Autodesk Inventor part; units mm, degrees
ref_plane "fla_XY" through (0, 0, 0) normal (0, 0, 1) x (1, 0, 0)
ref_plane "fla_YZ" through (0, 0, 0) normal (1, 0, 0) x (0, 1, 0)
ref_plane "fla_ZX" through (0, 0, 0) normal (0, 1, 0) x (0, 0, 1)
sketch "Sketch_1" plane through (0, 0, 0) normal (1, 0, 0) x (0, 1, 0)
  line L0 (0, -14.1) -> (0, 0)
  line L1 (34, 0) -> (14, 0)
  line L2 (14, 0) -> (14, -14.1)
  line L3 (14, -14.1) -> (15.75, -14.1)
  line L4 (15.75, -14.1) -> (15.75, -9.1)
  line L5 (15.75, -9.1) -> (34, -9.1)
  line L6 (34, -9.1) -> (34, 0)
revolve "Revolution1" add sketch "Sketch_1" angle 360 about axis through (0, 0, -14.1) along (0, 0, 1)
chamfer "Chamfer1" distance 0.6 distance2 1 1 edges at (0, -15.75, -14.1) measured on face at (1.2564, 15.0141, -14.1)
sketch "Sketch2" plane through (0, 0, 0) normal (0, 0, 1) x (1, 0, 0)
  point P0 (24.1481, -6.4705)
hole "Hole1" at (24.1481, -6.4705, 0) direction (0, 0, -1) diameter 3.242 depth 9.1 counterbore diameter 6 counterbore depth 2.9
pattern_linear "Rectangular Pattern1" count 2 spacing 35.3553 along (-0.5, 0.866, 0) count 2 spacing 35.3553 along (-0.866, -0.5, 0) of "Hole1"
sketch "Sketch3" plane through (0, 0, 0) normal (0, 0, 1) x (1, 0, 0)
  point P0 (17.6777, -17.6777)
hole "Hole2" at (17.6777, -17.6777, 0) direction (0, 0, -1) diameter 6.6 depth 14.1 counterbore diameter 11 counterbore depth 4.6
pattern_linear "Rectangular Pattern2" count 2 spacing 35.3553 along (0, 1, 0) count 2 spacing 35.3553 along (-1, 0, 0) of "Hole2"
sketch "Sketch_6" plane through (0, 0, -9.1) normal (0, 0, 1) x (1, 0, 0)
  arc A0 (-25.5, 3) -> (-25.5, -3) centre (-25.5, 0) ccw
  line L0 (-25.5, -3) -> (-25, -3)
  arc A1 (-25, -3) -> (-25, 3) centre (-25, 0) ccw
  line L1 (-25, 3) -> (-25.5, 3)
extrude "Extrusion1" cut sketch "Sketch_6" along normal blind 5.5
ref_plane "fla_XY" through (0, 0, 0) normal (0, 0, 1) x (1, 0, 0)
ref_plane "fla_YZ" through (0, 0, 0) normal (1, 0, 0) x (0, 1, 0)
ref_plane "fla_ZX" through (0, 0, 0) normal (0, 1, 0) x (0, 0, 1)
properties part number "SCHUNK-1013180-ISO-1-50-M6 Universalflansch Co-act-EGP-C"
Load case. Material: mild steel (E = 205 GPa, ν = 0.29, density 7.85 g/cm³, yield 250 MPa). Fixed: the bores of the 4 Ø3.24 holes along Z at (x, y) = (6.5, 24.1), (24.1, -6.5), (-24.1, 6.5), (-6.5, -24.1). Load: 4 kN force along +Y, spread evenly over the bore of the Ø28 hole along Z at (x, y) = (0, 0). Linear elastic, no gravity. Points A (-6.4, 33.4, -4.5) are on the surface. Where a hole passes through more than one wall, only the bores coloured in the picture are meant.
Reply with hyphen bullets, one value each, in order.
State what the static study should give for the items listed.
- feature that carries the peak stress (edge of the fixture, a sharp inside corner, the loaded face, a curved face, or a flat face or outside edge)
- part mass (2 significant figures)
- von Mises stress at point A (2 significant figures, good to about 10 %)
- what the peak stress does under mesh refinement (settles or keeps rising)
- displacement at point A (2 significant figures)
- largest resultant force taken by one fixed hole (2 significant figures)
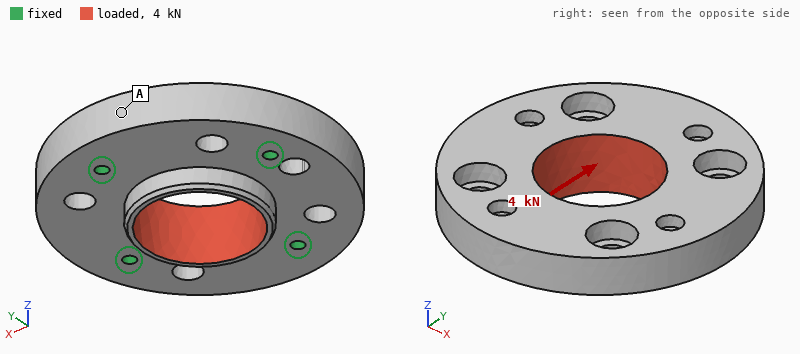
- edge of the fixture
- 200 g
- 3.6 MPa
- keeps rising
- 0.70 µm
- 1.1 kN
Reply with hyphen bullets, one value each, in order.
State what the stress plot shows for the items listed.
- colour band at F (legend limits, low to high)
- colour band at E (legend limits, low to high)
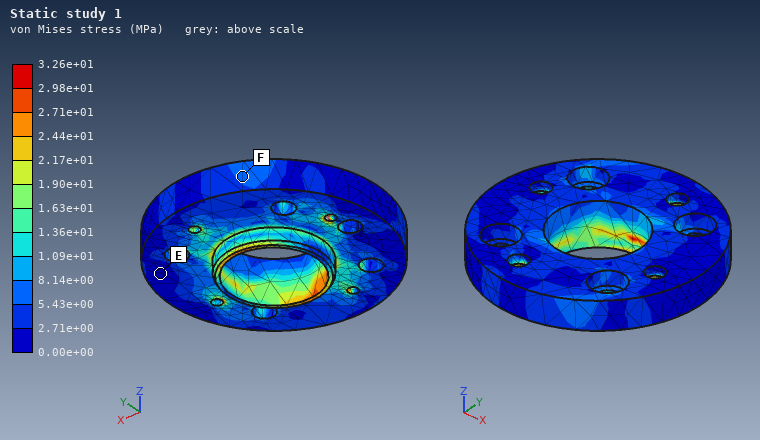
- 5.43e+00 to 8.14e+00 MPa
- 0.00e+00 to 2.71e+00 MPa
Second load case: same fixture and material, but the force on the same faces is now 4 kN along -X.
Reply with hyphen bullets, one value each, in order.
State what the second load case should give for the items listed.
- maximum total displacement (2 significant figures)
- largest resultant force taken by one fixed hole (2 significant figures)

- 3.3 µm
- 1.0 kN
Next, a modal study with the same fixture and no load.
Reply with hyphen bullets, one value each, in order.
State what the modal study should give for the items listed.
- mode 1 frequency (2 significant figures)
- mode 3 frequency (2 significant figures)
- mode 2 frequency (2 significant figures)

- 13 kHz
- 16 kHz
- 15 kHz
